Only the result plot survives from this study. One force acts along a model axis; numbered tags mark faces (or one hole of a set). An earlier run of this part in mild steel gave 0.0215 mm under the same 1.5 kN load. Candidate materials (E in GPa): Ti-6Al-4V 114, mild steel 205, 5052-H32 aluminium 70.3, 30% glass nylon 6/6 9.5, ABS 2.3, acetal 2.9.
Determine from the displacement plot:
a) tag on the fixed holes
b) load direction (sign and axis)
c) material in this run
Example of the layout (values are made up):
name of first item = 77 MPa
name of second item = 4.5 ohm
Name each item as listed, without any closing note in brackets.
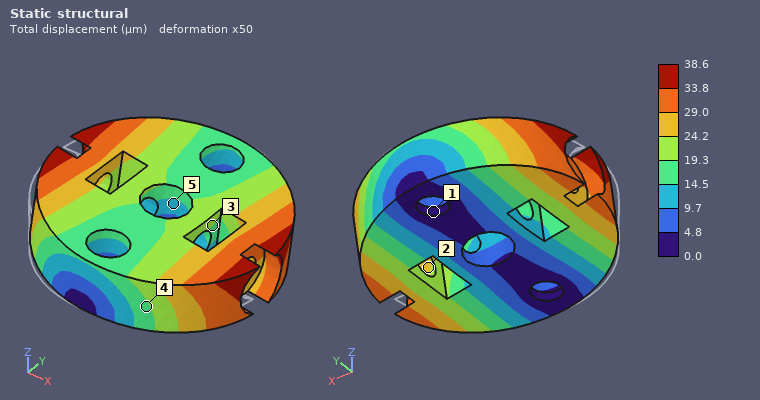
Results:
tag on the fixed holes = 1
load direction = +X
material in this run = Ti-6Al-4V
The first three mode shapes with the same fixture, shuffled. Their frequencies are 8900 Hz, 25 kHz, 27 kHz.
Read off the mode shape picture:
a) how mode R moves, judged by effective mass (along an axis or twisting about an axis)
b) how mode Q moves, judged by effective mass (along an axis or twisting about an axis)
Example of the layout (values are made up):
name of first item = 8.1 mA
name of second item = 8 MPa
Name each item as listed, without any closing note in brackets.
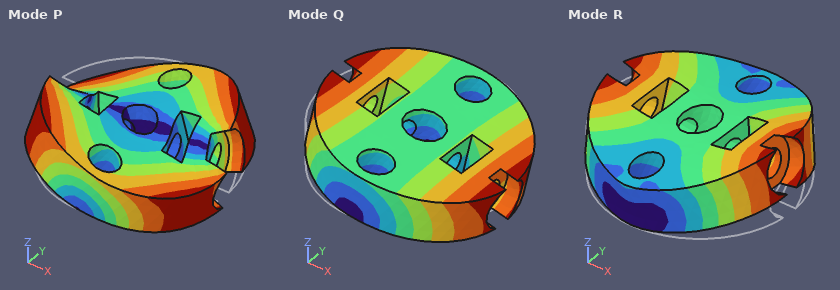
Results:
how mode R moves, judged by effective mass = along Z
how mode Q moves, judged by effective mass = along X
